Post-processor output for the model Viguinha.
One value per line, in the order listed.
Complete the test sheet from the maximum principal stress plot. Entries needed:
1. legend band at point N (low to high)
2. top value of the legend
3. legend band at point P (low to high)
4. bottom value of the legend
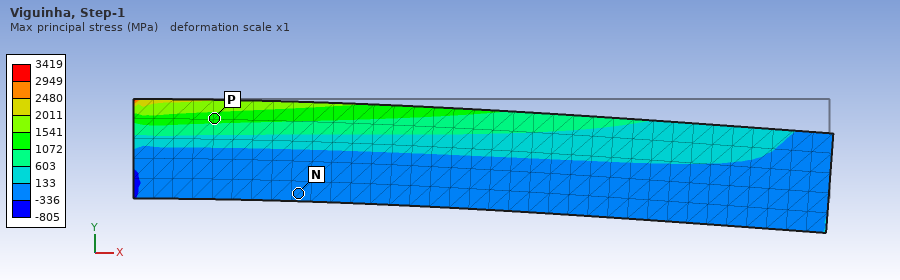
-336 to 133 MPa
3419 MPa
1072 to 1541 MPa
-805 MPa
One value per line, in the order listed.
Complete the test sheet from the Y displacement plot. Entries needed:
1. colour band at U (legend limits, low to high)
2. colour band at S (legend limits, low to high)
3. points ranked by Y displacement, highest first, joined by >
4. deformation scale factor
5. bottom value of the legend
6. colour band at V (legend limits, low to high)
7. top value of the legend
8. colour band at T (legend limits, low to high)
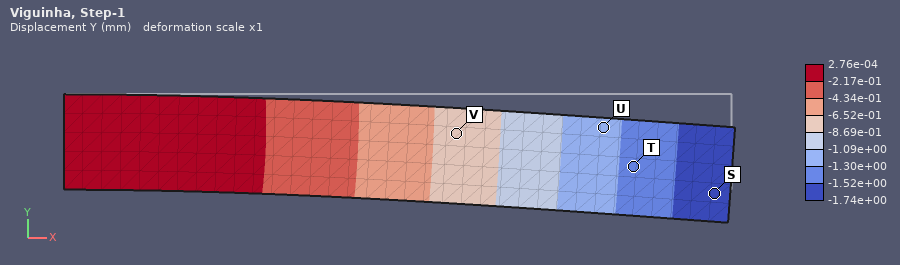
-1.30e+00 to -1.09e+00 mm
-1.74e+00 to -1.52e+00 mm
V > U > T > S
1
-1.74e+00 mm
-8.69e-01 to -6.52e-01 mm
2.76e-04 mm
-1.52e+00 to -1.30e+00 mm
